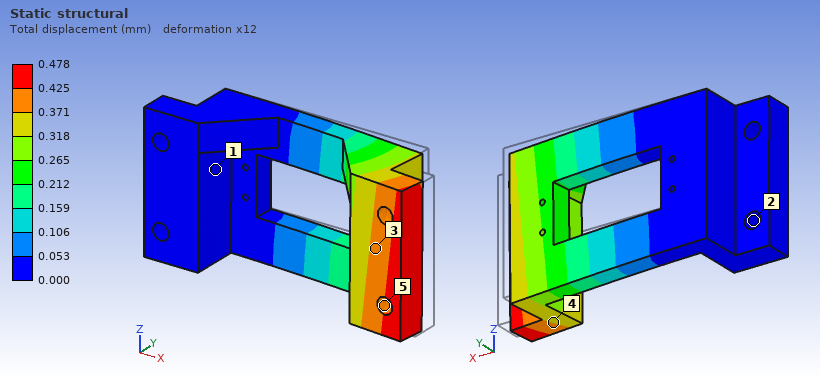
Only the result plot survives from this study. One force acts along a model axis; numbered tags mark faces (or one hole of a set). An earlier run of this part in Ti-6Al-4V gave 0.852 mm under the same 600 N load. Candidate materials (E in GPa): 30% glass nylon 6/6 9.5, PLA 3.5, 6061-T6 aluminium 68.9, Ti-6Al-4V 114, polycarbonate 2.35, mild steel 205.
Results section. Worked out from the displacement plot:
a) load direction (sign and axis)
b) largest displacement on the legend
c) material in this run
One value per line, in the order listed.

-Y
0.478 mm
mild steel
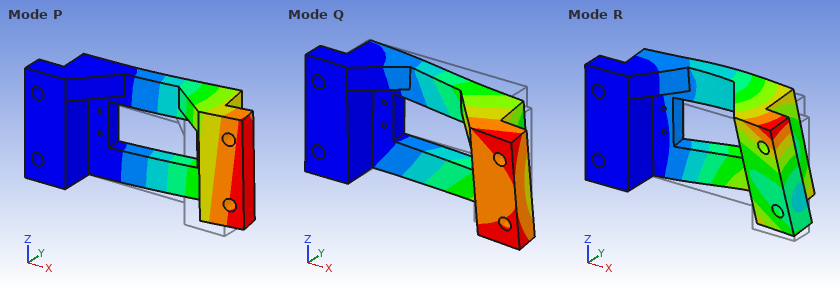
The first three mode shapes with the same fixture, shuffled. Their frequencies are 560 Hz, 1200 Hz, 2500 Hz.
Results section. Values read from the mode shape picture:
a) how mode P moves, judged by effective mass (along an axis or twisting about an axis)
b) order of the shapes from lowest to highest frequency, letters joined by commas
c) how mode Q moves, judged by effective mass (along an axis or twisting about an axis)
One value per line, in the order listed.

along Y
P, Q, R
along Z
